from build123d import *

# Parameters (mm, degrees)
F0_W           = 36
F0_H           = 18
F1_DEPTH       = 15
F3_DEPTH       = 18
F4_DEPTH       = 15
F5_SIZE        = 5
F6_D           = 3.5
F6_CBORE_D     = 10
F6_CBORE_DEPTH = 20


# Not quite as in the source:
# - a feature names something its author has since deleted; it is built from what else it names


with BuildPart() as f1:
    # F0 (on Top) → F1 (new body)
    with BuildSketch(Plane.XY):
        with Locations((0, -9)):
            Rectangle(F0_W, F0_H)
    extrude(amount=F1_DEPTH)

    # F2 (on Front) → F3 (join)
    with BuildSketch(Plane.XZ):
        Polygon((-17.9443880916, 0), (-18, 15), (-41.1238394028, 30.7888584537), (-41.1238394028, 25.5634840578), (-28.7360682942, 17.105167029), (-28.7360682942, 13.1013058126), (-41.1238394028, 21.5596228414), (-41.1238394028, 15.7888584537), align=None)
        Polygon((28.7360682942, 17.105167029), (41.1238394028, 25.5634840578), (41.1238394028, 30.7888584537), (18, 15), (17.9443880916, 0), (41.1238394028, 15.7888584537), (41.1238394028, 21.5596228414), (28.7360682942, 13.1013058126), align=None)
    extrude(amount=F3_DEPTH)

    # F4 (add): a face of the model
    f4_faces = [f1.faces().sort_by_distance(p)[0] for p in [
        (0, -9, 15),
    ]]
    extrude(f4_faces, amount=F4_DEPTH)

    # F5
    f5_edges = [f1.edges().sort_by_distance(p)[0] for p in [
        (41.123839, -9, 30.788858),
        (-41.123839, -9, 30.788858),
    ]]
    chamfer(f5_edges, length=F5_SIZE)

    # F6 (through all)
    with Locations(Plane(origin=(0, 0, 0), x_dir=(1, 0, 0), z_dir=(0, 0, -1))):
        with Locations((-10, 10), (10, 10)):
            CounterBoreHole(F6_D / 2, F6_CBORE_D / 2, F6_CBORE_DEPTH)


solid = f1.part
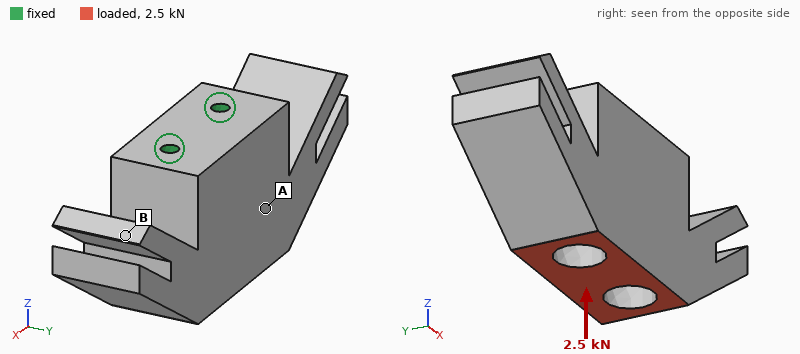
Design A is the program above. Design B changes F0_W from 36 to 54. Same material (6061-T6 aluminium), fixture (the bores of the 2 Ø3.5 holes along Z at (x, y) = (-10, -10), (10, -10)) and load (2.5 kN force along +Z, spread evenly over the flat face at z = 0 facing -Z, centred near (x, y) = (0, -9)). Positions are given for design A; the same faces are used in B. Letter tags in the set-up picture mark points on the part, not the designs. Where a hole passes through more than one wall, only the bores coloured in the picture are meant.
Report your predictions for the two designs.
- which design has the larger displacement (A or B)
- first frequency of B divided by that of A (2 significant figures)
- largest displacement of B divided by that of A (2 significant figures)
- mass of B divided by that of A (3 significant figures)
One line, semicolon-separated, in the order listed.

B; 0.99; 1.9; 1.04
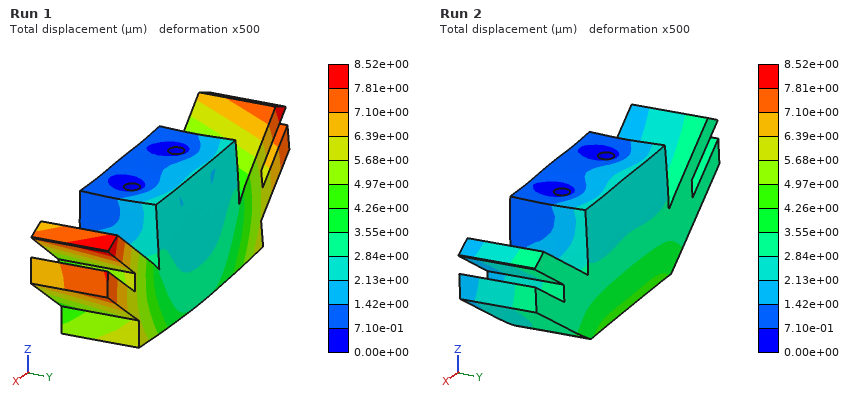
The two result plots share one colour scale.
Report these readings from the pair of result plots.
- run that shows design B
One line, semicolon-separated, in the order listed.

Run 1
